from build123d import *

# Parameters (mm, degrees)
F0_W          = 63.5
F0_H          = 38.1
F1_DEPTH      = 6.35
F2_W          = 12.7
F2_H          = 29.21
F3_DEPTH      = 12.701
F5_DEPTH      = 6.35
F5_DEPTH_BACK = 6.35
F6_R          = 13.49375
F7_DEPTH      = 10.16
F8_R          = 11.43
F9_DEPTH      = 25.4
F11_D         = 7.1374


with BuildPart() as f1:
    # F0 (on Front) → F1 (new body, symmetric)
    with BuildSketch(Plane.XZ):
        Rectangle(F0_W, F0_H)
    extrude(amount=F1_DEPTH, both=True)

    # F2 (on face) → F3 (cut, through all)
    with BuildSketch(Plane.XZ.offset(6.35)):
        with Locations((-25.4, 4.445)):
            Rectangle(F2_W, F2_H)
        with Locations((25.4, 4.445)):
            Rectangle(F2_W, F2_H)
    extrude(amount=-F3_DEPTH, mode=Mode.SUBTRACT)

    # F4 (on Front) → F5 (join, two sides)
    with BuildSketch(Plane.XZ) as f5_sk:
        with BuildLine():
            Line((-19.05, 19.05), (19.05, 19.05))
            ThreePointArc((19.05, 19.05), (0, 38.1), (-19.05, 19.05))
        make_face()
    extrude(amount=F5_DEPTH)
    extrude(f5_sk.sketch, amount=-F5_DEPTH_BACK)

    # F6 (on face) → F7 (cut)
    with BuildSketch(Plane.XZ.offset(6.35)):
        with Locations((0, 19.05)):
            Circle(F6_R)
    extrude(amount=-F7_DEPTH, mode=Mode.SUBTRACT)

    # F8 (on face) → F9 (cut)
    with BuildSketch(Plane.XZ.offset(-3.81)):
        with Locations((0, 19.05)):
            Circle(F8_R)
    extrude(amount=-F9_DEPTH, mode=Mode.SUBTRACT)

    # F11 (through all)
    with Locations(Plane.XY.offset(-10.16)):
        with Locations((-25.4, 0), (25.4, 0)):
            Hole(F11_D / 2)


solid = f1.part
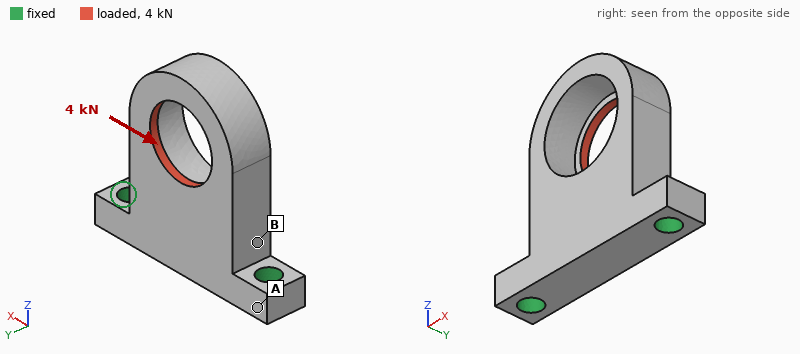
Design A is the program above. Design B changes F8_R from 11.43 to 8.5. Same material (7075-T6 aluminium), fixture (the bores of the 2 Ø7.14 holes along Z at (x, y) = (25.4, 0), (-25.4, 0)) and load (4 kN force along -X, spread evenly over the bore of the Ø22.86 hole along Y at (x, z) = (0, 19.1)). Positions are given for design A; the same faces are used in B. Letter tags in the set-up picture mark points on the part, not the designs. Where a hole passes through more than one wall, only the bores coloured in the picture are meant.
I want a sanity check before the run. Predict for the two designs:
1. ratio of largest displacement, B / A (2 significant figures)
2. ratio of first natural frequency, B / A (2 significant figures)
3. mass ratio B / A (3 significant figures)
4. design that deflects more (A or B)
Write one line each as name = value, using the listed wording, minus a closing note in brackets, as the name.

ratio of largest displacement, B / A = 0.75
ratio of first natural frequency, B / A = 0.98
mass ratio B / A = 1.02
design that deflects more = A
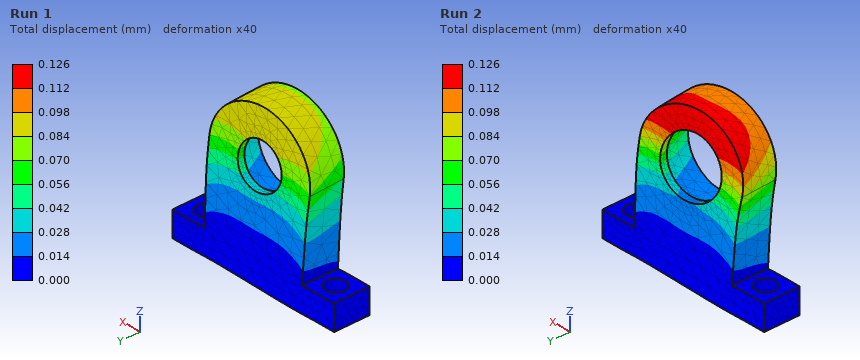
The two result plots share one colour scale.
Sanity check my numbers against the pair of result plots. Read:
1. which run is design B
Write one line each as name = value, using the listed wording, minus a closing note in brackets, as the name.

which run is design B = Run 1
